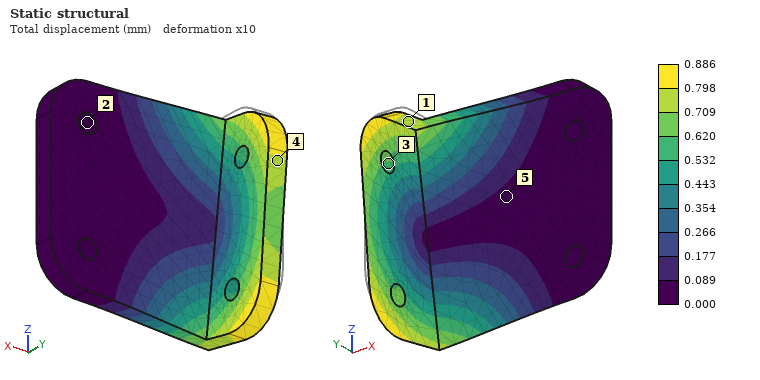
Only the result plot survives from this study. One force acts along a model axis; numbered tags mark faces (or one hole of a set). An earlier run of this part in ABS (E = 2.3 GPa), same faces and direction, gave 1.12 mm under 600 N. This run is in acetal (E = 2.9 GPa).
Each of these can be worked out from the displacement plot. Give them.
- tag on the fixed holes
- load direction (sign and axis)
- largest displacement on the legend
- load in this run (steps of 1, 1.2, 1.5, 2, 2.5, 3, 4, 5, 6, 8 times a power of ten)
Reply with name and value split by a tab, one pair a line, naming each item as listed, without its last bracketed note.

tag on the fixed holes	2
load direction	-Z
largest displacement on the legend	0.886 mm
load in this run	600 N
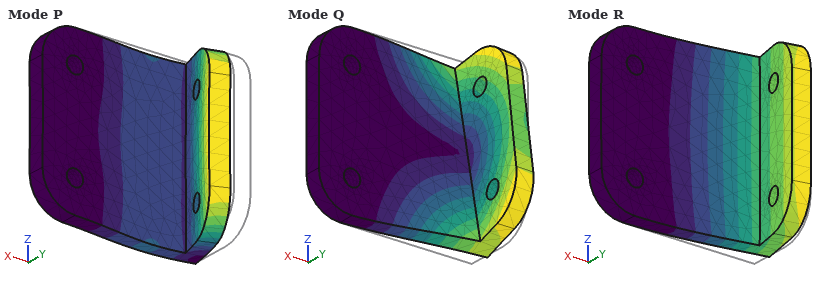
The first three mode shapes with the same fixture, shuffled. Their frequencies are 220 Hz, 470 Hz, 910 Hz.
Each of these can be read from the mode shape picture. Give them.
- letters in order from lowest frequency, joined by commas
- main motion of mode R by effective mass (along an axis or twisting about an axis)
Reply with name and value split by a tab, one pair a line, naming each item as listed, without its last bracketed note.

letters in order from lowest frequency, joined by commas	R, Q, P
main motion of mode R by effective mass	along Y
